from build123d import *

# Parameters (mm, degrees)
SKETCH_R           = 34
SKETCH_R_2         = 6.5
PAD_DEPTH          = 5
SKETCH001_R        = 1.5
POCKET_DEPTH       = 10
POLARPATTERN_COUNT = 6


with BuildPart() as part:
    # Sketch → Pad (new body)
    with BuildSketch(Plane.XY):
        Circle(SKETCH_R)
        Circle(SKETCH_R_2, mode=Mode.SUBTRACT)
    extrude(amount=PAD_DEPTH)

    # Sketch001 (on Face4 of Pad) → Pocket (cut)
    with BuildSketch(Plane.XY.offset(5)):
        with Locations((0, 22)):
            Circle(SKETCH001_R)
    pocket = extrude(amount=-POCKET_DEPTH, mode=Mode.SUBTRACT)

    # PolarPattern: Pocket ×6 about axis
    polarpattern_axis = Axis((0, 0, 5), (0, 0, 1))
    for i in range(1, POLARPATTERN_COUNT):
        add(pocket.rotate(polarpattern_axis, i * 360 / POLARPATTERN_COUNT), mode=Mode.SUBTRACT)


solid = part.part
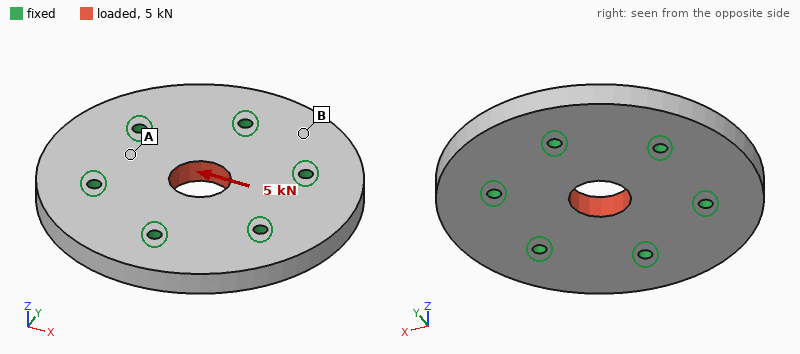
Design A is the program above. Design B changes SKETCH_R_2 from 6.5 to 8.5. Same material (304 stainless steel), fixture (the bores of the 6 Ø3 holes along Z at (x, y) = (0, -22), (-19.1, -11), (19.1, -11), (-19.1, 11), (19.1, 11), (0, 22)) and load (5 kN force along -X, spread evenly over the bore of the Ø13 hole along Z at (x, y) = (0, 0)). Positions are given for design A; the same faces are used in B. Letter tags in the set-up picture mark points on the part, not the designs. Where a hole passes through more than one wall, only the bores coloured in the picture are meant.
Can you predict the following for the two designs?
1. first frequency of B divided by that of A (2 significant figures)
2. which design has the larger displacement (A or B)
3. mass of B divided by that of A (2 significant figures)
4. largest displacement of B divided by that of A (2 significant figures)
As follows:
1.0
A
0.97
0.82
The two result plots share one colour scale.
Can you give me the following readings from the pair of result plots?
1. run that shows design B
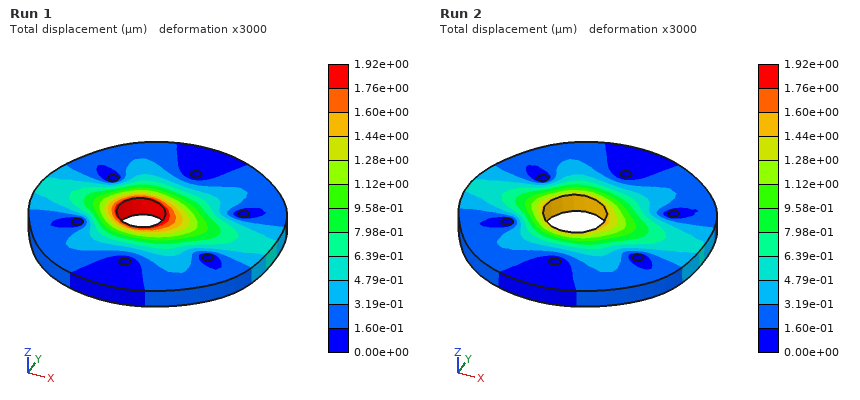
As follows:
Run 2
